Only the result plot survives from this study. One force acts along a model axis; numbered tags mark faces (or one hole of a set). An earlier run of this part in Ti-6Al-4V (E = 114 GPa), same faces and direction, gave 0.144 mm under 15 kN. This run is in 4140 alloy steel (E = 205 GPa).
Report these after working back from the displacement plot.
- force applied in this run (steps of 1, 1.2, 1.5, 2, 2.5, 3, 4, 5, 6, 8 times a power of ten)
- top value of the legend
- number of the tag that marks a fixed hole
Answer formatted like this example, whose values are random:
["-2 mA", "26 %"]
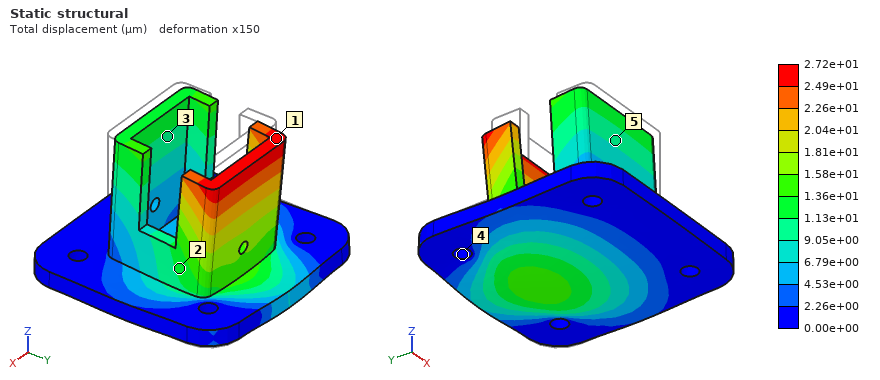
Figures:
["5 kN", "2.72e+01 µm", "4"]
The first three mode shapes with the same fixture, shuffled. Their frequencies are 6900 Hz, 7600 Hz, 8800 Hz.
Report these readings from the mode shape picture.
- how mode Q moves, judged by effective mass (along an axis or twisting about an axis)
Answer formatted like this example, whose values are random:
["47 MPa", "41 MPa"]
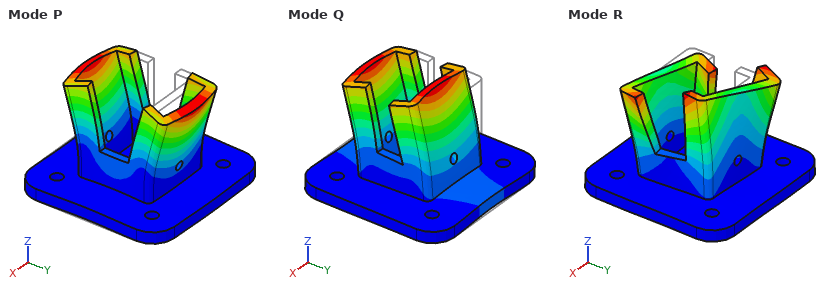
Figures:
["along Y"]
